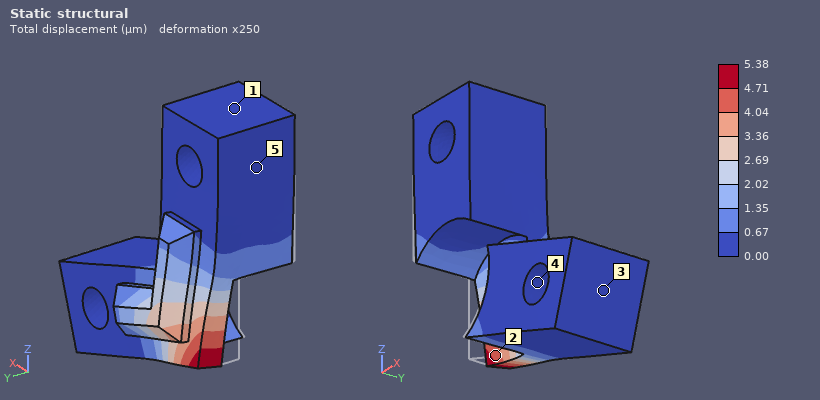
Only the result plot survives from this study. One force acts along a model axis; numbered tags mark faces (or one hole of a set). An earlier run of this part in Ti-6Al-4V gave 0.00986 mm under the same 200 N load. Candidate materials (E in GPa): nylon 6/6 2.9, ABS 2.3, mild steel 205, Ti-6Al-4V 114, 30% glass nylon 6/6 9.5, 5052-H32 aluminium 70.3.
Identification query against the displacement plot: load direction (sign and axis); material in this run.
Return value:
+Y
mild steel
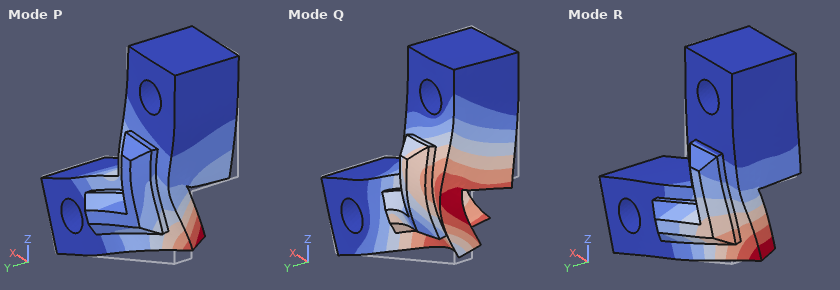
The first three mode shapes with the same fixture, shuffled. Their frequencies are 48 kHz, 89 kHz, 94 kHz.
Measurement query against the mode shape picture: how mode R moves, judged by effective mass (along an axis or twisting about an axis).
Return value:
along Y
